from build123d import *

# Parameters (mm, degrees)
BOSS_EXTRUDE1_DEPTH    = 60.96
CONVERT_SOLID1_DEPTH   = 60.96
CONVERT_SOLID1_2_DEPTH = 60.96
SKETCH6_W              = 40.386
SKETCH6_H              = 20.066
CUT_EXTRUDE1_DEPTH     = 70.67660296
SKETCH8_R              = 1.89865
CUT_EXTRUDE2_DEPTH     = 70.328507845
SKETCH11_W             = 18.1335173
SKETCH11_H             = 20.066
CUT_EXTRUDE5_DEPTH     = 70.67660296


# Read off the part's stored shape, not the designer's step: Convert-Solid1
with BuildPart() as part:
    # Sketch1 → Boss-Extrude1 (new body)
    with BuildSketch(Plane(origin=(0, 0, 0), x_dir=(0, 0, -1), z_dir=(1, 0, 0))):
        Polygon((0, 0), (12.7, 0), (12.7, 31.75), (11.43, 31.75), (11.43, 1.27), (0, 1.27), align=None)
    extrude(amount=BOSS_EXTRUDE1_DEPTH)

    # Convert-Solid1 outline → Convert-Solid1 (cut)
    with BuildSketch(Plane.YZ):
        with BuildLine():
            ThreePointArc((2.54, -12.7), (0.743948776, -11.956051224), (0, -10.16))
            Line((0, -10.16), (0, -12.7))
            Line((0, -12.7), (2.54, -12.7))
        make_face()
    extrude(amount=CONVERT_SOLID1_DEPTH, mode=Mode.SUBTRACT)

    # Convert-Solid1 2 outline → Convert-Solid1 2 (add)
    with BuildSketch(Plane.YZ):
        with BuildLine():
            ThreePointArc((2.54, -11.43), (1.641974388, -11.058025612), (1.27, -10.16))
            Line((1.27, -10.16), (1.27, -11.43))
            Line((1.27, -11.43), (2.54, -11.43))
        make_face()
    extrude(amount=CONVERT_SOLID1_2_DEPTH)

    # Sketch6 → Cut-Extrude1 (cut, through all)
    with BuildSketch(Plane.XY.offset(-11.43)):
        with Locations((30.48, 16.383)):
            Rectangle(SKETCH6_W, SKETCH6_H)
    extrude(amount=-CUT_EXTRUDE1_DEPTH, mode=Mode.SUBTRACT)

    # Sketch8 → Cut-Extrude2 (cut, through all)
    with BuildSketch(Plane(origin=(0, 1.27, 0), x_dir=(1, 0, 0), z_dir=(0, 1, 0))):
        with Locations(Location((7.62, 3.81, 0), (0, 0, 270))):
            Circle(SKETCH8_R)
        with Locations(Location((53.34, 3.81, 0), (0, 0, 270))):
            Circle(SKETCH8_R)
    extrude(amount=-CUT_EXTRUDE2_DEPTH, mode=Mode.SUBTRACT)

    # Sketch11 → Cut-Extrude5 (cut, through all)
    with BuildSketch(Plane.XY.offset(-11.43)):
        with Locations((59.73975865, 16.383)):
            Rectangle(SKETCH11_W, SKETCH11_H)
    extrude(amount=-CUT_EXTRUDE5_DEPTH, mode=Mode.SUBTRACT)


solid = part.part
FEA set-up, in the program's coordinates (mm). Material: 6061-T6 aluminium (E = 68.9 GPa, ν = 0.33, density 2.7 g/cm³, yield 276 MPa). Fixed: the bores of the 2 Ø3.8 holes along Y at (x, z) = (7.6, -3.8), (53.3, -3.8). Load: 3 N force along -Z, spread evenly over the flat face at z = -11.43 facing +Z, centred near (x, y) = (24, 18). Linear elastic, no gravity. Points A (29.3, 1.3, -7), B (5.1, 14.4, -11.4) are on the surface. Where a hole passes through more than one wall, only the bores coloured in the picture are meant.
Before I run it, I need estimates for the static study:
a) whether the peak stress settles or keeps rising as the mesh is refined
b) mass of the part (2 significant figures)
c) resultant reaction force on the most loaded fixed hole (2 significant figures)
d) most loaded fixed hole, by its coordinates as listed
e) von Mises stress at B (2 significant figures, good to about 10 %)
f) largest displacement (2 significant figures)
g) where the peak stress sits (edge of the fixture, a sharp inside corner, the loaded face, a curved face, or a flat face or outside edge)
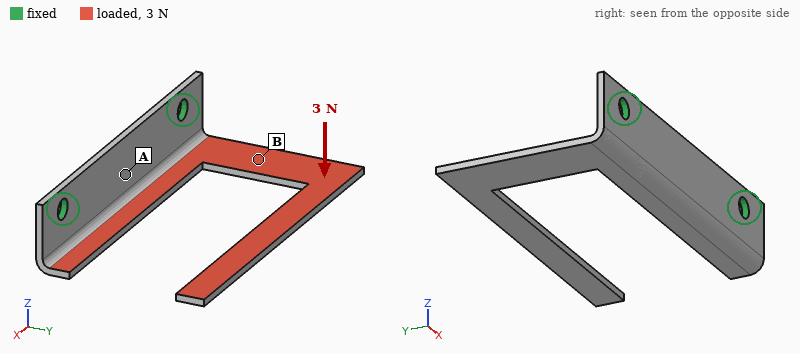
keeps rising
5.3 g
2.4 N
(7.6, -3.8)
13 MPa
0.71 mm
a sharp inside corner
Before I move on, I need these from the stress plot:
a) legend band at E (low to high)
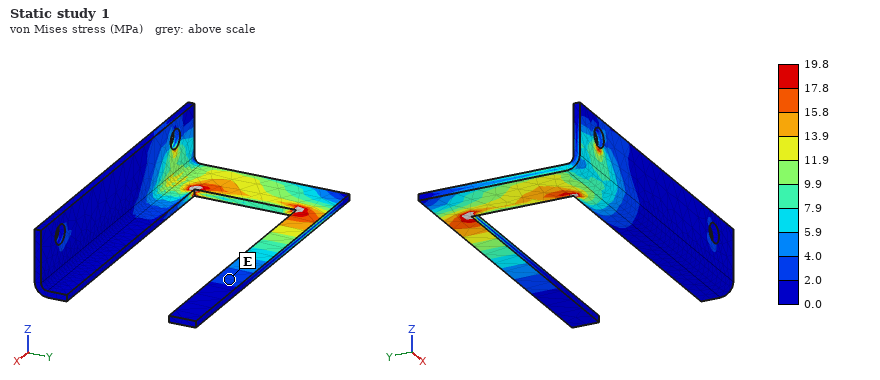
2.0 to 4.0 MPa
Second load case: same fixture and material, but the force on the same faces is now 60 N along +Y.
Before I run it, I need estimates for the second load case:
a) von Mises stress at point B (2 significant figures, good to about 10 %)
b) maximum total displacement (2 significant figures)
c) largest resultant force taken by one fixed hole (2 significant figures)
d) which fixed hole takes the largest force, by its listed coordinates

11 MPa
0.67 mm
50 N
(7.6, -3.8)
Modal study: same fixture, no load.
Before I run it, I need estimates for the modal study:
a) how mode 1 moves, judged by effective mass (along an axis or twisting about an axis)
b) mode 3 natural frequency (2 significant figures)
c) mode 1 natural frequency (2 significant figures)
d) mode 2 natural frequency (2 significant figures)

along Z
1100 Hz
260 Hz
740 Hz
